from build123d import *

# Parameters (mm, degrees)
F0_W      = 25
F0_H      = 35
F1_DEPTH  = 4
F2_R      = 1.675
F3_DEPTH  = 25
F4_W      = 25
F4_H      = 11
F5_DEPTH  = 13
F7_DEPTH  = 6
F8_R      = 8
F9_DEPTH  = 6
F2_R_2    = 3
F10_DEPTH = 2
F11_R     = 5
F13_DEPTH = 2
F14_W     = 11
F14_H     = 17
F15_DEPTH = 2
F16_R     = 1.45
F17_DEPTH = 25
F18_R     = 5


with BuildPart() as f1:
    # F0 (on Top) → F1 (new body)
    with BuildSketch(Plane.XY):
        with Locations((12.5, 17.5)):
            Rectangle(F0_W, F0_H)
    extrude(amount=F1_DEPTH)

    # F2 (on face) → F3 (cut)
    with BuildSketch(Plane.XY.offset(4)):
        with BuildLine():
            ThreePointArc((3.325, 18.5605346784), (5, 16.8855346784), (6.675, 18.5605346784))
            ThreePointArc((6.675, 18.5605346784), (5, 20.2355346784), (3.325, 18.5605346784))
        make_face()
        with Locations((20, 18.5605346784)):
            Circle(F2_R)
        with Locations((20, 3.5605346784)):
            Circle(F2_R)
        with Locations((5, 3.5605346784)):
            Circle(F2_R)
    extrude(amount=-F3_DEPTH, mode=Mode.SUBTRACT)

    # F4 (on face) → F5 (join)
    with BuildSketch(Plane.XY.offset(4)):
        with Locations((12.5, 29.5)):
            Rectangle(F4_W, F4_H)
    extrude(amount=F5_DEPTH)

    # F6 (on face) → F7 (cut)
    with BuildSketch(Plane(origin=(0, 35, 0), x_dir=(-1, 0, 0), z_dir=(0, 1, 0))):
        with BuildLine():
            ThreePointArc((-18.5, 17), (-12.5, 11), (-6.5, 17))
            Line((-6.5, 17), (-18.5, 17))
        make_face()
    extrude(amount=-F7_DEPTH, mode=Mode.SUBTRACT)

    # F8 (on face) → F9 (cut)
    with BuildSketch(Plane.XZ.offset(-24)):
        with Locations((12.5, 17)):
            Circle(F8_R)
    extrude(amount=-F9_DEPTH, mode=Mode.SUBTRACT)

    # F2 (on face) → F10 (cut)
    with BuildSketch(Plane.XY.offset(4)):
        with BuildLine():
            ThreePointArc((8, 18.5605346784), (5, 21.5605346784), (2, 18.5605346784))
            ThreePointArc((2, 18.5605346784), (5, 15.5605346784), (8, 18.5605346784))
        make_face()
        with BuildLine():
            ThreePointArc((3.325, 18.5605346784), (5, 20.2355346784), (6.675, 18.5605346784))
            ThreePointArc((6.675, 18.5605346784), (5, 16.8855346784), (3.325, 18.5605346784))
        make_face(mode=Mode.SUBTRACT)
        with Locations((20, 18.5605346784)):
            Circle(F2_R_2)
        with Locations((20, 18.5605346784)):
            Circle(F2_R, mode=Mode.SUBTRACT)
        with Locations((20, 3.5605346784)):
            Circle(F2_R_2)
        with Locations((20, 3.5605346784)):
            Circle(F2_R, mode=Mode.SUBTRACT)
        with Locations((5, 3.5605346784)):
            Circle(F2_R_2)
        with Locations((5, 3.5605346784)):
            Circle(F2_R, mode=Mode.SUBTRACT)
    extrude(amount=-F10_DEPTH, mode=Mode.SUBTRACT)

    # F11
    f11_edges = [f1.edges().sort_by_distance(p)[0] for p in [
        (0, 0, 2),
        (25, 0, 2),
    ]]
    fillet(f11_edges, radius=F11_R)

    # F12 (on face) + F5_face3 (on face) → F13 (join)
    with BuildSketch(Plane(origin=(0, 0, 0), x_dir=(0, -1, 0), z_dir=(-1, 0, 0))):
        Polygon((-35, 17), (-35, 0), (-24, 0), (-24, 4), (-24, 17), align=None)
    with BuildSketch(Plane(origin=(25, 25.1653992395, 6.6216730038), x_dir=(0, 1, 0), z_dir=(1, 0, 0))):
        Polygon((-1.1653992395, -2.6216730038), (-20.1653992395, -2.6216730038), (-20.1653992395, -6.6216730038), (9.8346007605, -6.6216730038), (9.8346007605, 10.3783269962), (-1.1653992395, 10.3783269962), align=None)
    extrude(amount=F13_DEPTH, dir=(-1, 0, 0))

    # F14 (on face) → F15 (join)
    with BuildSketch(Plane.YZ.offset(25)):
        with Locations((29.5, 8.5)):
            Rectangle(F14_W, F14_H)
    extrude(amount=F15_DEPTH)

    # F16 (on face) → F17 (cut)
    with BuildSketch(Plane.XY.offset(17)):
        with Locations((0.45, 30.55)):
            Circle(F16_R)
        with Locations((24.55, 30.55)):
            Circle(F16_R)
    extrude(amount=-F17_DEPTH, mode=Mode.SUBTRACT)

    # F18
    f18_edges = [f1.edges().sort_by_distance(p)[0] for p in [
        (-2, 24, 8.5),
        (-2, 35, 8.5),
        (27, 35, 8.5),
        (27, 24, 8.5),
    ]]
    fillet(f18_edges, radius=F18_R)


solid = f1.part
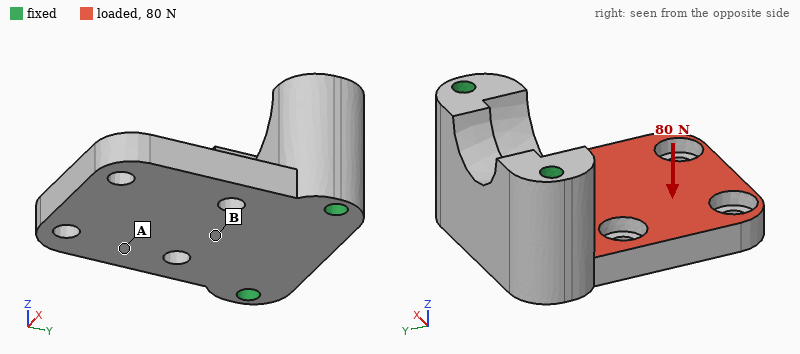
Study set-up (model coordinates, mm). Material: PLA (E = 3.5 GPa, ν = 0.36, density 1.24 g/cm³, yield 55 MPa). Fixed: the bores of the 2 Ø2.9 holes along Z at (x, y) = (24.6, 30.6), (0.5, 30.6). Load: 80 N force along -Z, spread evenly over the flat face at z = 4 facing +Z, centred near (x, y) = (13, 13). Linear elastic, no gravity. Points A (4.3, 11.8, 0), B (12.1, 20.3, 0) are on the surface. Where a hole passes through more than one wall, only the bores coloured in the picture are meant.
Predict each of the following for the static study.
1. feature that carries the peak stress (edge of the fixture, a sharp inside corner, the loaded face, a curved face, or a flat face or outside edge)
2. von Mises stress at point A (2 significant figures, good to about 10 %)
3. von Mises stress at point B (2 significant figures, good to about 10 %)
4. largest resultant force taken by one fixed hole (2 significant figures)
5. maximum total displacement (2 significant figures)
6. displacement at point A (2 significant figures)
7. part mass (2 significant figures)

the loaded face
3.1 MPa
11 MPa
41 N
0.49 mm
0.21 mm
7.5 g
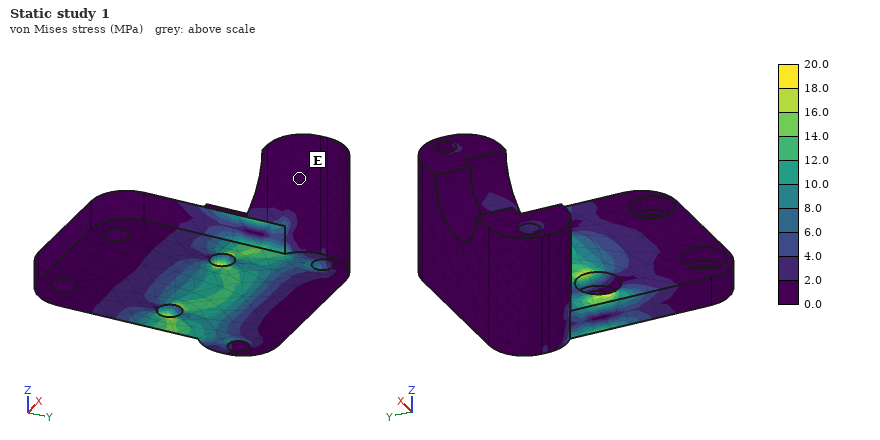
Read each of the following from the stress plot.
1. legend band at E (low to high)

0.0 to 2.0 MPa
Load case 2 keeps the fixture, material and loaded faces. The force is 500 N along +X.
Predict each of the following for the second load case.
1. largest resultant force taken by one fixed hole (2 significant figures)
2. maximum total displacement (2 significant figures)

440 N
0.34 mm
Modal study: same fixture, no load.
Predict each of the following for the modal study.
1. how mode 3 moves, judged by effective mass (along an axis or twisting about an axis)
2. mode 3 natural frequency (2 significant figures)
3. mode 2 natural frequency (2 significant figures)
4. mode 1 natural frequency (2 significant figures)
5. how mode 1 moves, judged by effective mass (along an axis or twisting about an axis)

along X
5900 Hz
3900 Hz
1600 Hz
along Z
